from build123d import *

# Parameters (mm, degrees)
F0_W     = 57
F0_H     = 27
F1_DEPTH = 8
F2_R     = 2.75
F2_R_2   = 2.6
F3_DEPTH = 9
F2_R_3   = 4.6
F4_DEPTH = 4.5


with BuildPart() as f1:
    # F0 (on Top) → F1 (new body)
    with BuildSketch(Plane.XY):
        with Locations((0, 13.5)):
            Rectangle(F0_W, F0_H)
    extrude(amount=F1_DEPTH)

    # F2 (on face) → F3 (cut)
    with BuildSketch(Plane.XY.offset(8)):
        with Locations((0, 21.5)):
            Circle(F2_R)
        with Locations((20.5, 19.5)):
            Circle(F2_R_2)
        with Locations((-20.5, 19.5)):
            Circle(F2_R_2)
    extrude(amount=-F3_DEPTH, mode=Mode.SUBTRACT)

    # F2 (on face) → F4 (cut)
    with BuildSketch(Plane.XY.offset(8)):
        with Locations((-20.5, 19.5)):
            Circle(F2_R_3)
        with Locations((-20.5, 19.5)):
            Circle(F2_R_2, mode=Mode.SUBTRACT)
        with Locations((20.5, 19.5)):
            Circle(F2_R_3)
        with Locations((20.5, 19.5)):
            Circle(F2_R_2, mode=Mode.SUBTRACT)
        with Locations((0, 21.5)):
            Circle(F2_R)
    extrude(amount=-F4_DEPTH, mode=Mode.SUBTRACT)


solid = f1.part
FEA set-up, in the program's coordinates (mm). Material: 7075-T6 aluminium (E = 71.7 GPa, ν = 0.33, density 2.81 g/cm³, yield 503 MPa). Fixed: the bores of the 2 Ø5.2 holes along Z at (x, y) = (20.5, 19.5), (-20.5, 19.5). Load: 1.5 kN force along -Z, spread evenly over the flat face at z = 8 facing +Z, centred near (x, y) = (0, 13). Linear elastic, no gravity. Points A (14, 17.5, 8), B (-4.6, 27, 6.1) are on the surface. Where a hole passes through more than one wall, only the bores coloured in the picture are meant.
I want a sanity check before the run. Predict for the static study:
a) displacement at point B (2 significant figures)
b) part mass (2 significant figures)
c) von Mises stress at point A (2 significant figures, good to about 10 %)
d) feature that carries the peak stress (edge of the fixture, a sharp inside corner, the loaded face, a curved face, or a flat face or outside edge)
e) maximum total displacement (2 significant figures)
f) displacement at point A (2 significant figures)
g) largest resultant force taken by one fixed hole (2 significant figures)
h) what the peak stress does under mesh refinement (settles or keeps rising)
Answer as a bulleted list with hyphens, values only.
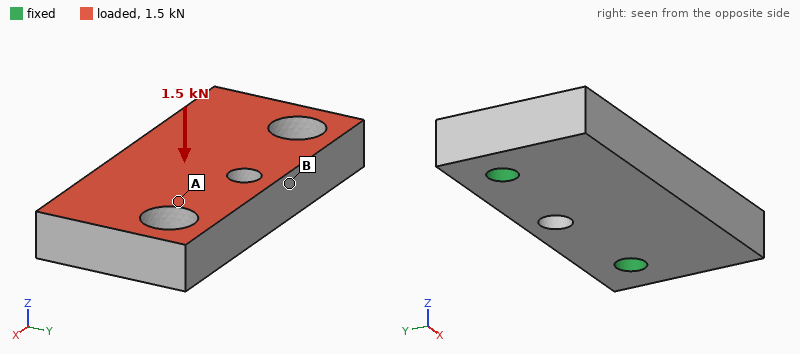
- 6.2 µm
- 32 g
- 21 MPa
- edge of the fixture
- 38 µm
- 10 µm
- 800 N
- keeps rising
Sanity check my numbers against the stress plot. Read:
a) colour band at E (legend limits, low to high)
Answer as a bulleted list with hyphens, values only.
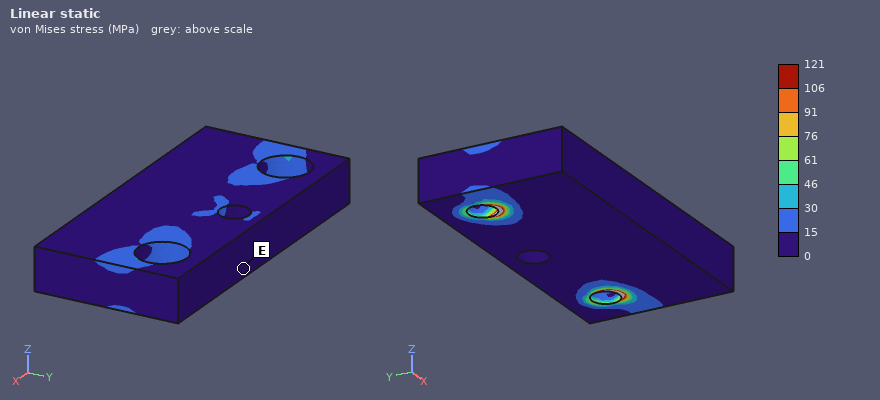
- 0 to 15 MPa
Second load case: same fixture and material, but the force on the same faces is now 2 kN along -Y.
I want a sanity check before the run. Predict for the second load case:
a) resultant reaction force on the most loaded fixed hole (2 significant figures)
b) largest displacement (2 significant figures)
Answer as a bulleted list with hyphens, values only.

- 1.0 kN
- 41 µm
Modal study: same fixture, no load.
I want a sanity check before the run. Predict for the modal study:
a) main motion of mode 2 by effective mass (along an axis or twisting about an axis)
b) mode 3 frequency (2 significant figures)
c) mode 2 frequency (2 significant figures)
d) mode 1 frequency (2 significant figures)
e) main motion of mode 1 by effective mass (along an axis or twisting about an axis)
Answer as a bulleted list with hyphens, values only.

- twisting about Y
- 15 kHz
- 13 kHz
- 6800 Hz
- along Z
